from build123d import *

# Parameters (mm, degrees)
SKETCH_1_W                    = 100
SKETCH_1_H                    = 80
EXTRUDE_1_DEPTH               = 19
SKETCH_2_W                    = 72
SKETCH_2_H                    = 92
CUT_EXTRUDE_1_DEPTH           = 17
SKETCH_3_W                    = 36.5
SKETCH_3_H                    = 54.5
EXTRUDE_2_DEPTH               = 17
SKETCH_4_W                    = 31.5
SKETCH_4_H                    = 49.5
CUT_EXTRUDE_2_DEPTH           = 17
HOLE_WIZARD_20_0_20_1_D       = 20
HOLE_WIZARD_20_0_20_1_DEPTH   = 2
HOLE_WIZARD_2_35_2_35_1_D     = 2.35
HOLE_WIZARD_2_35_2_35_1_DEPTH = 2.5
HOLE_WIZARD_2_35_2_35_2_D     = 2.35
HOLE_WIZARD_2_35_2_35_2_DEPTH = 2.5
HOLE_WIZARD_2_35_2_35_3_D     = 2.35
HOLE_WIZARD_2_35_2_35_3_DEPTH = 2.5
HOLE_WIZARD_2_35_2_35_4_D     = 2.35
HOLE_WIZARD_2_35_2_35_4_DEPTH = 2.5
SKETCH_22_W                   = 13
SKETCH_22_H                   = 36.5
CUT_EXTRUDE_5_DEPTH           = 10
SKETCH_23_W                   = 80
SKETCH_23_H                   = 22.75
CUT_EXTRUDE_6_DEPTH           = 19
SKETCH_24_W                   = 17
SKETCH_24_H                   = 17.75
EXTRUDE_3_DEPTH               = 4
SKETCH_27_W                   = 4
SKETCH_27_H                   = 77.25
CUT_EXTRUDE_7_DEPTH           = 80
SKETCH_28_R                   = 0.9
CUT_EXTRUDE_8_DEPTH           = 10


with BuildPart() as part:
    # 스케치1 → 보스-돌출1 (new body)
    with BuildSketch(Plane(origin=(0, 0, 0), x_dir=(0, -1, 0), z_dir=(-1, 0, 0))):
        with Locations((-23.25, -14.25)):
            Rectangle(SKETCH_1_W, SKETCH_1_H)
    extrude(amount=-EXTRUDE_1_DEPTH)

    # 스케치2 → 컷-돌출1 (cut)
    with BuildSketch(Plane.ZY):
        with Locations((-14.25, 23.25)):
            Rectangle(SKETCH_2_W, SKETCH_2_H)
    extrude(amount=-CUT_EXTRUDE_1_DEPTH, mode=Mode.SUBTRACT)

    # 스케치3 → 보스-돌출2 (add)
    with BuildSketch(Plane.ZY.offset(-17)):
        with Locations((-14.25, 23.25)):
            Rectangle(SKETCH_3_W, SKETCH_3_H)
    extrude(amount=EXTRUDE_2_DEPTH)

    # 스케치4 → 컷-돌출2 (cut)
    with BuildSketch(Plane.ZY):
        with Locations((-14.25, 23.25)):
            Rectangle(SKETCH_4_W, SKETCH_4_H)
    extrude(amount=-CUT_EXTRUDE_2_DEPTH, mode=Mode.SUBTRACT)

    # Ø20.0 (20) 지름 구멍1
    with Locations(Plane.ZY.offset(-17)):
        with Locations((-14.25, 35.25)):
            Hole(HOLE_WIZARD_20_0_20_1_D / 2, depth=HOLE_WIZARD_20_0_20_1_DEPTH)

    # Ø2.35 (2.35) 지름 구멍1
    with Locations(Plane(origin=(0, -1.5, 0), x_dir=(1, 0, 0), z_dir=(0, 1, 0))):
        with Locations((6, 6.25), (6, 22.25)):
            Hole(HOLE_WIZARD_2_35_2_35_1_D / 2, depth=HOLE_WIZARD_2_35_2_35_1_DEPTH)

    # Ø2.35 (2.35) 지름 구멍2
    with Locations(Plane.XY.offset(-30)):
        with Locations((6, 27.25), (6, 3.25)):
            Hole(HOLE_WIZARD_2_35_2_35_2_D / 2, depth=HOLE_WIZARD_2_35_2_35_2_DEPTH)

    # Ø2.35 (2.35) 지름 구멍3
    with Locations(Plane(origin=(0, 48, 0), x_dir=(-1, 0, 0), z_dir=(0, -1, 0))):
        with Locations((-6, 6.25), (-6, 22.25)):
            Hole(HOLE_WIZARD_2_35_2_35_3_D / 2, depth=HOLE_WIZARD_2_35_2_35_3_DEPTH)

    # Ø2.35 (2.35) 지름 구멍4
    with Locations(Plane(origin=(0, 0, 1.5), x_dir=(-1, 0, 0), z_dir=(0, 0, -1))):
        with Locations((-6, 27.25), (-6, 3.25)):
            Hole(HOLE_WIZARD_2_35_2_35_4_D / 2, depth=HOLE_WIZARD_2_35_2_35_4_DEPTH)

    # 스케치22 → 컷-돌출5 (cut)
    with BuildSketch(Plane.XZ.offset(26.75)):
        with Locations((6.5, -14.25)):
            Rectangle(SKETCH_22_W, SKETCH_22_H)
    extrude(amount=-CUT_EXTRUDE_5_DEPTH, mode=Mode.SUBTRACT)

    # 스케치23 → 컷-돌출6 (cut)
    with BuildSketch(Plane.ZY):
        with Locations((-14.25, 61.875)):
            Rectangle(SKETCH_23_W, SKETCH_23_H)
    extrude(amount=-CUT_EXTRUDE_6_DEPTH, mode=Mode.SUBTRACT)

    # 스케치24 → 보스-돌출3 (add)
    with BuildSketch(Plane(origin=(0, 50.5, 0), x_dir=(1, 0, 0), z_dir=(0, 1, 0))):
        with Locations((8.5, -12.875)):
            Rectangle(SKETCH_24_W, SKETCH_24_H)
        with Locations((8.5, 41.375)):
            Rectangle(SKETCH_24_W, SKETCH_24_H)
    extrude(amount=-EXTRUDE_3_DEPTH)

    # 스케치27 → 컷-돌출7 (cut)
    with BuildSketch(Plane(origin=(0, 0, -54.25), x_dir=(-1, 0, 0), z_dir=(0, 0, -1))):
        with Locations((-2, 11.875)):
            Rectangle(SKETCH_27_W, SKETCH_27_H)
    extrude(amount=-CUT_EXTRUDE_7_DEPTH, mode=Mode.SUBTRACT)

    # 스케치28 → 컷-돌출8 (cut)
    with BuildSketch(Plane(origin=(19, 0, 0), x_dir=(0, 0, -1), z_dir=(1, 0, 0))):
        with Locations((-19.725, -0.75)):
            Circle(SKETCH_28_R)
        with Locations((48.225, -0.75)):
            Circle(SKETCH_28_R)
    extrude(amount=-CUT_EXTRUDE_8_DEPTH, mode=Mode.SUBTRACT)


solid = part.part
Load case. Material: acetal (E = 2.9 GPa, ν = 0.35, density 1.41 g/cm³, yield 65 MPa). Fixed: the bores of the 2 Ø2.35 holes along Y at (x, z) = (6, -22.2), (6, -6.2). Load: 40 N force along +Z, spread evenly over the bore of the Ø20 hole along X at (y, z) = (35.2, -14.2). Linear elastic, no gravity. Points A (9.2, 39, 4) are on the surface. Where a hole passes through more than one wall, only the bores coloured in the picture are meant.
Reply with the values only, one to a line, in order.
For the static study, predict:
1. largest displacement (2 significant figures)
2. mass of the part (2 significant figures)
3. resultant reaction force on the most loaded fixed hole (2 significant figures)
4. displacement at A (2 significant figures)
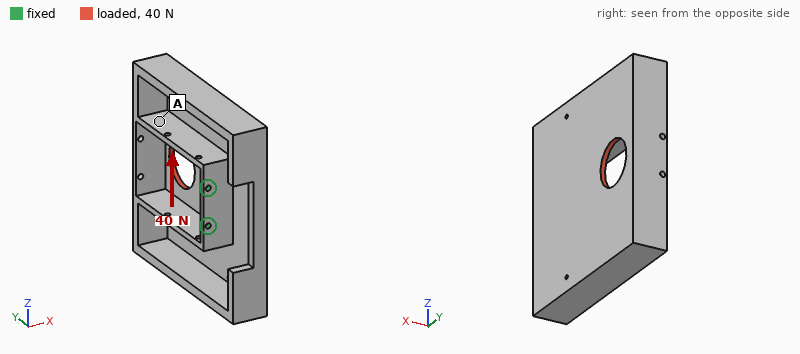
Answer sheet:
1.1 mm
42 g
76 N
0.76 mm
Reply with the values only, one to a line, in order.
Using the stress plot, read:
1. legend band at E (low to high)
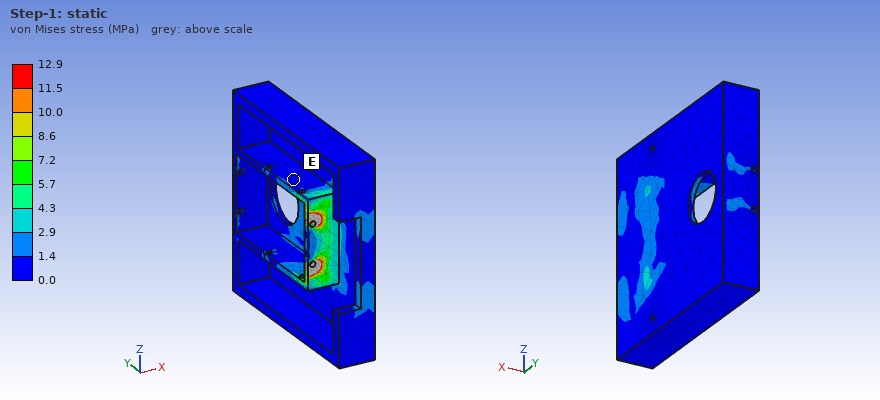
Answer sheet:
0.0 to 1.4 MPa
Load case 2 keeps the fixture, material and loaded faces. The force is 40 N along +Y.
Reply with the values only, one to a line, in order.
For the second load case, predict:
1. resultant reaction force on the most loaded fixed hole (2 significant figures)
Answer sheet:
20 N
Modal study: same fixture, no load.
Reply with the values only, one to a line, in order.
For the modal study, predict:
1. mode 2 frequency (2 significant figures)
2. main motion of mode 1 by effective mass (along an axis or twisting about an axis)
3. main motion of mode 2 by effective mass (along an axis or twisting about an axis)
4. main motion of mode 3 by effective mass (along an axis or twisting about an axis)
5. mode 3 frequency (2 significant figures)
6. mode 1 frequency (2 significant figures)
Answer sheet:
180 Hz
along X
along Z
twisting about Y
310 Hz
110 Hz
